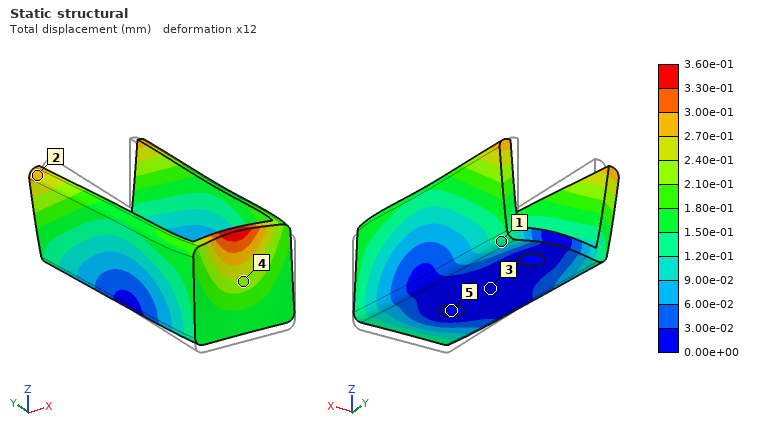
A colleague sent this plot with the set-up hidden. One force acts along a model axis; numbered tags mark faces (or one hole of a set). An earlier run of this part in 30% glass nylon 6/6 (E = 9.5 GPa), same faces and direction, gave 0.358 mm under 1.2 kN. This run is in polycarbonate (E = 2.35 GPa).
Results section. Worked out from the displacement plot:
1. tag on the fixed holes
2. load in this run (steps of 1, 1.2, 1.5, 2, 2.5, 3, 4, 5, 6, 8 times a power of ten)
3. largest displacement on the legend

5
300 N
3.60e-01 mm
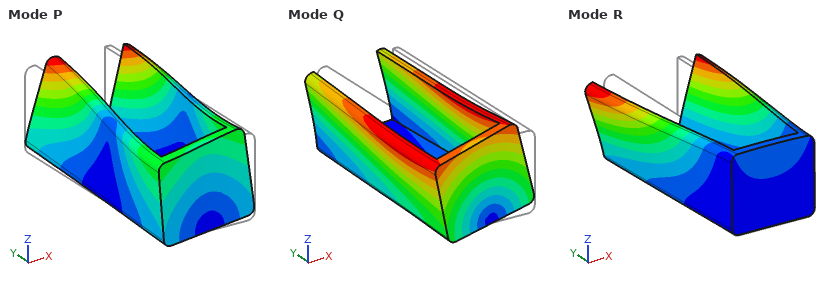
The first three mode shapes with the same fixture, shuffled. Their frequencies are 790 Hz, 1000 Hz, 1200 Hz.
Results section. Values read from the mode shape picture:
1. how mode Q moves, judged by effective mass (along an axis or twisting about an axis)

along X
